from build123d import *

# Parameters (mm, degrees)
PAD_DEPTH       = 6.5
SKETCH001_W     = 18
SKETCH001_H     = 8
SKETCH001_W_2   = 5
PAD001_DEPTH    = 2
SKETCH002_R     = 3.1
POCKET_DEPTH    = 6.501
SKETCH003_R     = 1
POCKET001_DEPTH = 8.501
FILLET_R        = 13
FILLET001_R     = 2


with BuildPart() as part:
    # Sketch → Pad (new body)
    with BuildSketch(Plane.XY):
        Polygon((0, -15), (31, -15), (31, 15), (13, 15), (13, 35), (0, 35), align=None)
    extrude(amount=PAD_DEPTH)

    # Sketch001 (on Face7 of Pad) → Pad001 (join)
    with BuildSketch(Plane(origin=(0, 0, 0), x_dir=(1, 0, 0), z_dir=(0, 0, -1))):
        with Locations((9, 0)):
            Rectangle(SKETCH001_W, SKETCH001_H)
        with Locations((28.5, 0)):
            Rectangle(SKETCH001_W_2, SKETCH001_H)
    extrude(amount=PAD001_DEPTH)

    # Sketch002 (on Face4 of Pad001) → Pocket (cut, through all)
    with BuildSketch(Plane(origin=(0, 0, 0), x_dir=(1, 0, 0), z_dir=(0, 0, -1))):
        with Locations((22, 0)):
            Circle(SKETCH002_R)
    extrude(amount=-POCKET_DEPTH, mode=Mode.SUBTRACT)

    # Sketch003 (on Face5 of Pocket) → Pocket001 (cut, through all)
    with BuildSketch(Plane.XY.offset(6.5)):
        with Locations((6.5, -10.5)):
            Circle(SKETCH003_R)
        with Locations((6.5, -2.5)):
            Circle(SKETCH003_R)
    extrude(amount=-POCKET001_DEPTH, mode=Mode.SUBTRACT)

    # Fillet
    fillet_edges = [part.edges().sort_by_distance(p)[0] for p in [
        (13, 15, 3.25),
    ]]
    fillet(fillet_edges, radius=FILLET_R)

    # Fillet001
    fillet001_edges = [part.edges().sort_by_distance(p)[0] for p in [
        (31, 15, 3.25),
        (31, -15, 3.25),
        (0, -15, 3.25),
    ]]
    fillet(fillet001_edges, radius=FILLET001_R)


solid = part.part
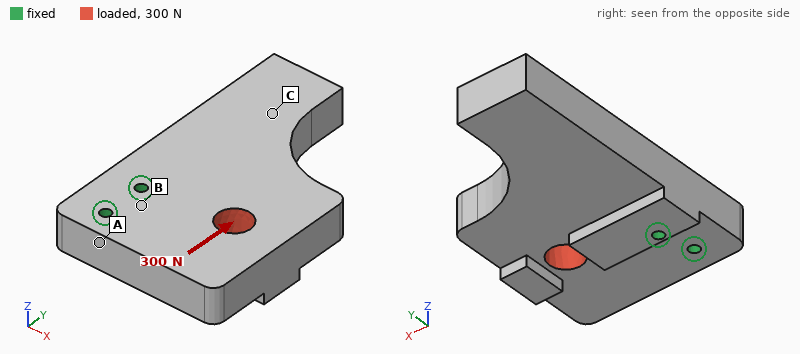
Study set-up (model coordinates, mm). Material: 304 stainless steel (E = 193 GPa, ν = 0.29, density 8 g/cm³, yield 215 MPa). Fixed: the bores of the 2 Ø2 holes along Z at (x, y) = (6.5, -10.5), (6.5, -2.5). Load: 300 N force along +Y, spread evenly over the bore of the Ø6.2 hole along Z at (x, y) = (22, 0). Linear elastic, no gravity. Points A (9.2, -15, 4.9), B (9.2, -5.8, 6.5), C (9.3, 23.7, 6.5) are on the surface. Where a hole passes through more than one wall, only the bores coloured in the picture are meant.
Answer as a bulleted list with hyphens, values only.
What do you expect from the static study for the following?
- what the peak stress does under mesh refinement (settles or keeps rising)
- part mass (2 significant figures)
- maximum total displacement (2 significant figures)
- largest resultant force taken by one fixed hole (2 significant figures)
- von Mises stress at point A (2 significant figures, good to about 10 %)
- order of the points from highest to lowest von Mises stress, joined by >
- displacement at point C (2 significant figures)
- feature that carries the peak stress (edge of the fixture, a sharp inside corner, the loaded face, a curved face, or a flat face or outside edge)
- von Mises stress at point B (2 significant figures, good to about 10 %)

- keeps rising
- 65 g
- 3.8 µm
- 510 N
- 6.1 MPa
- B > A > C
- 2.6 µm
- edge of the fixture
- 9.1 MPa
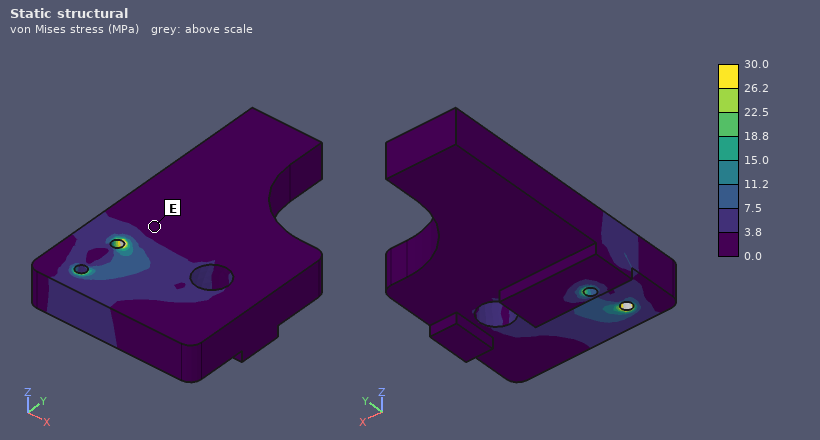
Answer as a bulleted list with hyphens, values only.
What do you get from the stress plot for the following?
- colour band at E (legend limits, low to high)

- 0.0 to 3.8 MPa
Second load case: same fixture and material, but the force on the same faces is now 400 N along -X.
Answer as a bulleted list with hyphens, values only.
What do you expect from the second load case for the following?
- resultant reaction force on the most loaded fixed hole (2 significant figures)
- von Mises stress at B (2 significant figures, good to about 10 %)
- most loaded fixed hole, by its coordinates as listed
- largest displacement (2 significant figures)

- 470 N
- 4.0 MPa
- (6.5, -2.5)
- 2.1 µm
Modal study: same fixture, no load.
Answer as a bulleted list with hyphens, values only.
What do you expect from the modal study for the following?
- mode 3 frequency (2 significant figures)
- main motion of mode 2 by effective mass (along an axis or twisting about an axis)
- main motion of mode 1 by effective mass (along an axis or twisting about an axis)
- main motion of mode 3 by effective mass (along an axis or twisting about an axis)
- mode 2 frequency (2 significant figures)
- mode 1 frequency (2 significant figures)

- 7400 Hz
- along X
- along Z
- along Z
- 6500 Hz
- 4400 Hz
